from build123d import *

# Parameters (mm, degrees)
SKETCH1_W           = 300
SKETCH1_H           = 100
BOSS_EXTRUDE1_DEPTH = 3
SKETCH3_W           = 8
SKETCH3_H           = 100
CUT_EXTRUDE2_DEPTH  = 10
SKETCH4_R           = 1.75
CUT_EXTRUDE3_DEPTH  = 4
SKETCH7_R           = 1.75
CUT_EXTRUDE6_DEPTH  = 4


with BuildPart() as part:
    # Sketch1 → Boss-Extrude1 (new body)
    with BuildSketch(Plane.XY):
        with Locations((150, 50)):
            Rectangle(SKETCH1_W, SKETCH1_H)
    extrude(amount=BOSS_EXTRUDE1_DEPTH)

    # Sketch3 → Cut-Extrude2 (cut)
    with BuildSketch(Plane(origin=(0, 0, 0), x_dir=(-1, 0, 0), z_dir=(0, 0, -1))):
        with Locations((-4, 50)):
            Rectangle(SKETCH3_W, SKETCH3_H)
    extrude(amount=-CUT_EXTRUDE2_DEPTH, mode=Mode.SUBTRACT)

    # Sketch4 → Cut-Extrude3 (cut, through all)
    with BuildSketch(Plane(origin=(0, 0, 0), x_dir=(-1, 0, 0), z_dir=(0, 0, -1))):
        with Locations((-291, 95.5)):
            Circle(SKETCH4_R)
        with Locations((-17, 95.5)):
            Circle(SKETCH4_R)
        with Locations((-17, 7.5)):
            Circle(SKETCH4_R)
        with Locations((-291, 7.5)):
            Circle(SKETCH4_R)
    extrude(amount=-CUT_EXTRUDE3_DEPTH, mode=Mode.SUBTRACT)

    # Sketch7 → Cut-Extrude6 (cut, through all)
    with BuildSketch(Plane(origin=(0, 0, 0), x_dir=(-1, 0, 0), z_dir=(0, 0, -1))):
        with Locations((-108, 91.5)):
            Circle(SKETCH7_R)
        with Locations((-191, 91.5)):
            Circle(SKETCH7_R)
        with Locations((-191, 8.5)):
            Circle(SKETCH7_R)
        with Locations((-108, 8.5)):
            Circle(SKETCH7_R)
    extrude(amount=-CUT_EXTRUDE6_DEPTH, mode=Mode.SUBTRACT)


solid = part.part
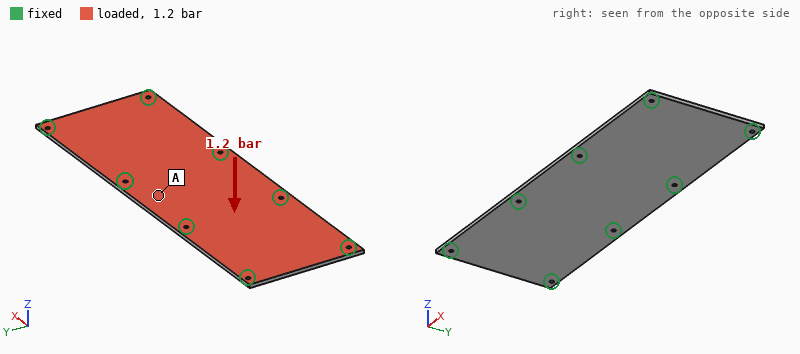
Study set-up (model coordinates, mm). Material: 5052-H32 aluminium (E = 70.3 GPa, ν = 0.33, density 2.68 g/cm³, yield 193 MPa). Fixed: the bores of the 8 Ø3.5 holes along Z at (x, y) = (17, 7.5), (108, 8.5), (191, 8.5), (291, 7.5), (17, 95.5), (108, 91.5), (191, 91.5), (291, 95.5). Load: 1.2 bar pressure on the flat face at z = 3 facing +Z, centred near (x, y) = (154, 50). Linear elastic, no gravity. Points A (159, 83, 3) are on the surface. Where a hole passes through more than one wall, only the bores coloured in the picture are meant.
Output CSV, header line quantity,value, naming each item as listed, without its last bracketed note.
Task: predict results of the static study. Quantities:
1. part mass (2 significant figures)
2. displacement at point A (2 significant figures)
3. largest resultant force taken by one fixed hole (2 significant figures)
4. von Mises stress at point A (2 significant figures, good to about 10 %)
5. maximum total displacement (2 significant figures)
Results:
quantity,value
part mass,230 g
displacement at point A,0.12 mm
largest resultant force taken by one fixed hole,570 N
von Mises stress at point A,18 MPa
maximum total displacement,0.40 mm
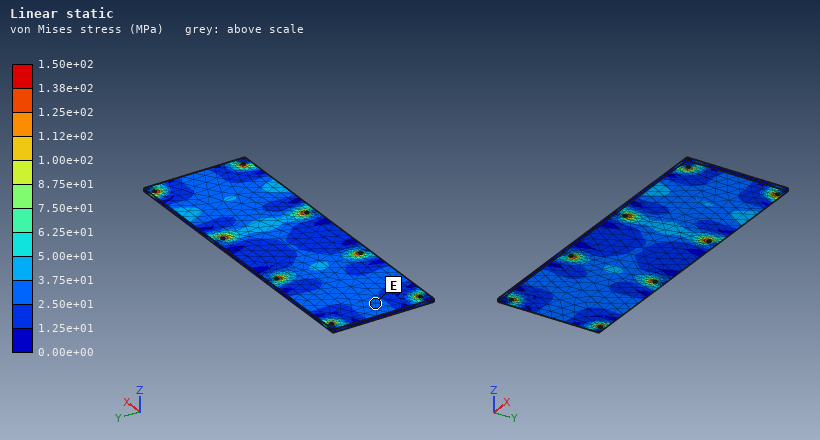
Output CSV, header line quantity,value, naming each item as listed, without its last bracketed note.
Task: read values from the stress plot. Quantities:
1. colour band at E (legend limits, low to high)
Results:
quantity,value
colour band at E,2.50e+01 to 3.75e+01 MPa
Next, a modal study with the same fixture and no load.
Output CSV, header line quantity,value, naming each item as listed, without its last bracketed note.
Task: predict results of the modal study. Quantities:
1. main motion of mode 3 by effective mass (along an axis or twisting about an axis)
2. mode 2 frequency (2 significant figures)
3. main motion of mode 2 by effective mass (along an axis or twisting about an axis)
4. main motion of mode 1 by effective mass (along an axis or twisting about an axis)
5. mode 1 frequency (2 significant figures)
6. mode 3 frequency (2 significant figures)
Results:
quantity,value
main motion of mode 3 by effective mass,along Z
mode 2 frequency,1300 Hz
main motion of mode 2 by effective mass,along Z
main motion of mode 1 by effective mass,along Z
mode 1 frequency,1200 Hz
mode 3 frequency,1500 Hz
